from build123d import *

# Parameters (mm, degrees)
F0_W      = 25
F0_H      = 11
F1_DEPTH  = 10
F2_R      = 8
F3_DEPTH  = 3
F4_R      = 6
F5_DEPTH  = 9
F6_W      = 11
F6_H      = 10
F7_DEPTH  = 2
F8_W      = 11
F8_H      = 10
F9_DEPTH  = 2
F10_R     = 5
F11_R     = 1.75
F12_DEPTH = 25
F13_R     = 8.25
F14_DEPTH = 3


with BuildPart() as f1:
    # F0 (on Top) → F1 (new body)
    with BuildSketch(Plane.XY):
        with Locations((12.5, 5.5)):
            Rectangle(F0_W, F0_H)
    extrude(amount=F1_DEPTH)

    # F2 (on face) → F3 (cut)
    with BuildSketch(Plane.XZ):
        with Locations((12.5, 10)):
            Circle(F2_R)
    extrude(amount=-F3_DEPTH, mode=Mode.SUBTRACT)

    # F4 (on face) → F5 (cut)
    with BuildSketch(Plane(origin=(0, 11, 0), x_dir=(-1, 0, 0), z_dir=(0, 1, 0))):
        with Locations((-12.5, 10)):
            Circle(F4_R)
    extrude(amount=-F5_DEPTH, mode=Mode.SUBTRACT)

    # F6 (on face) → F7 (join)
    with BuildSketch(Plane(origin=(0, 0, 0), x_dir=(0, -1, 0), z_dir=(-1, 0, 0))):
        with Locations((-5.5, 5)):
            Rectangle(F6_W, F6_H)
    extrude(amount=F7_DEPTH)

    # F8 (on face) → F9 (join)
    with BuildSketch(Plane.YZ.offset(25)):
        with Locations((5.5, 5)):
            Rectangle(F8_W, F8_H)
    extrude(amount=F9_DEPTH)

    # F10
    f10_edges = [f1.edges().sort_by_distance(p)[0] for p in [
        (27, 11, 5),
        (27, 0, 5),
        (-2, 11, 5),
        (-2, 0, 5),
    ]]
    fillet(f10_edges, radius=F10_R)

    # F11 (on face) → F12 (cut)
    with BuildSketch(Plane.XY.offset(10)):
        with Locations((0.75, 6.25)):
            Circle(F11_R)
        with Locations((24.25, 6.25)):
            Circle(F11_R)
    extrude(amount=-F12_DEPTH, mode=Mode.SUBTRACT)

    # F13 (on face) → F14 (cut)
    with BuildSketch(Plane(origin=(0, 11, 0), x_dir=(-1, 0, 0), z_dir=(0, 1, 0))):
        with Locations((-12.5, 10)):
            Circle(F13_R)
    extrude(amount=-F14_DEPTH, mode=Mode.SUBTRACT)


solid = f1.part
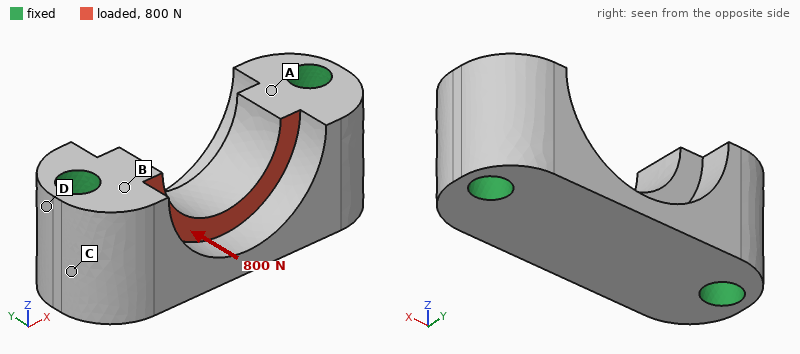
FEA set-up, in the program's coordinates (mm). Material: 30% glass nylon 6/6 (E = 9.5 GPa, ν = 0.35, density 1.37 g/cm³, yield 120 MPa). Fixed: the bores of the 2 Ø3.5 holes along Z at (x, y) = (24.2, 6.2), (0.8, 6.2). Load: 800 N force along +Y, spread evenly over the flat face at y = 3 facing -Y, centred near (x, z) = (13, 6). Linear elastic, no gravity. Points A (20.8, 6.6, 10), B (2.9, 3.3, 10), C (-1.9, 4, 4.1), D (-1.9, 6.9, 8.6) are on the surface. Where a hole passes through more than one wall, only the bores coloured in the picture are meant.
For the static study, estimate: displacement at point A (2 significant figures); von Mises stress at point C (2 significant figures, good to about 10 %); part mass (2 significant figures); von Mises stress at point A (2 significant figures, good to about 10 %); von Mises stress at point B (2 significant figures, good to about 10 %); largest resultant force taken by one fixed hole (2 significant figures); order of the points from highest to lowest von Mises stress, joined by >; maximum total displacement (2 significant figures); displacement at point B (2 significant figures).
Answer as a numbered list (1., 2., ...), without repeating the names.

1. 6.8 µm
2. 5.9 MPa
3. 2.6 g
4. 14 MPa
5. 9.5 MPa
6. 410 N
7. A > B > C > D
8. 31 µm
9. 6.1 µm
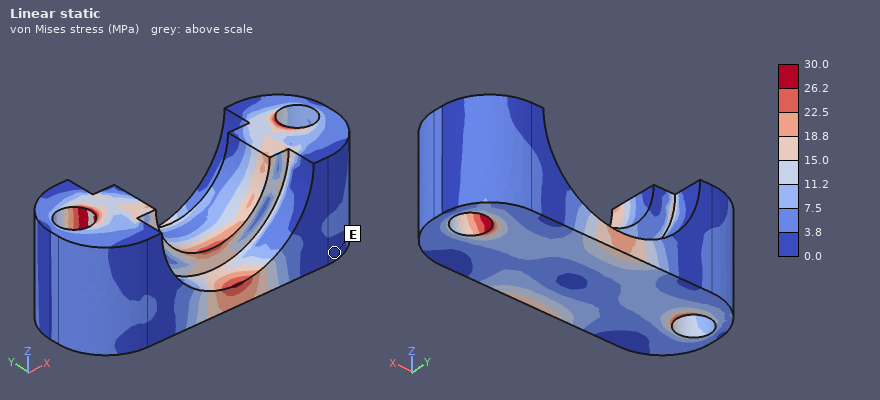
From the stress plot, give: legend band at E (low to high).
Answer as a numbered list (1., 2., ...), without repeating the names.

1. 0.0 to 3.8 MPa
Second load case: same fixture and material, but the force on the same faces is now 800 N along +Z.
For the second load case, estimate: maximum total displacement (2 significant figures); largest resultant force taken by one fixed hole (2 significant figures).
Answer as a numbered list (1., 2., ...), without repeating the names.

1. 40 µm
2. 420 N
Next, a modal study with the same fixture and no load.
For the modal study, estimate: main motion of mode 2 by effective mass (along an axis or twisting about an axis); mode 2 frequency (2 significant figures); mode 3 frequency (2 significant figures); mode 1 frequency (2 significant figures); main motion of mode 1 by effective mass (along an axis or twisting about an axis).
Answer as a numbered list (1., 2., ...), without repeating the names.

1. along Z
2. 34 kHz
3. 44 kHz
4. 27 kHz
5. along Y
